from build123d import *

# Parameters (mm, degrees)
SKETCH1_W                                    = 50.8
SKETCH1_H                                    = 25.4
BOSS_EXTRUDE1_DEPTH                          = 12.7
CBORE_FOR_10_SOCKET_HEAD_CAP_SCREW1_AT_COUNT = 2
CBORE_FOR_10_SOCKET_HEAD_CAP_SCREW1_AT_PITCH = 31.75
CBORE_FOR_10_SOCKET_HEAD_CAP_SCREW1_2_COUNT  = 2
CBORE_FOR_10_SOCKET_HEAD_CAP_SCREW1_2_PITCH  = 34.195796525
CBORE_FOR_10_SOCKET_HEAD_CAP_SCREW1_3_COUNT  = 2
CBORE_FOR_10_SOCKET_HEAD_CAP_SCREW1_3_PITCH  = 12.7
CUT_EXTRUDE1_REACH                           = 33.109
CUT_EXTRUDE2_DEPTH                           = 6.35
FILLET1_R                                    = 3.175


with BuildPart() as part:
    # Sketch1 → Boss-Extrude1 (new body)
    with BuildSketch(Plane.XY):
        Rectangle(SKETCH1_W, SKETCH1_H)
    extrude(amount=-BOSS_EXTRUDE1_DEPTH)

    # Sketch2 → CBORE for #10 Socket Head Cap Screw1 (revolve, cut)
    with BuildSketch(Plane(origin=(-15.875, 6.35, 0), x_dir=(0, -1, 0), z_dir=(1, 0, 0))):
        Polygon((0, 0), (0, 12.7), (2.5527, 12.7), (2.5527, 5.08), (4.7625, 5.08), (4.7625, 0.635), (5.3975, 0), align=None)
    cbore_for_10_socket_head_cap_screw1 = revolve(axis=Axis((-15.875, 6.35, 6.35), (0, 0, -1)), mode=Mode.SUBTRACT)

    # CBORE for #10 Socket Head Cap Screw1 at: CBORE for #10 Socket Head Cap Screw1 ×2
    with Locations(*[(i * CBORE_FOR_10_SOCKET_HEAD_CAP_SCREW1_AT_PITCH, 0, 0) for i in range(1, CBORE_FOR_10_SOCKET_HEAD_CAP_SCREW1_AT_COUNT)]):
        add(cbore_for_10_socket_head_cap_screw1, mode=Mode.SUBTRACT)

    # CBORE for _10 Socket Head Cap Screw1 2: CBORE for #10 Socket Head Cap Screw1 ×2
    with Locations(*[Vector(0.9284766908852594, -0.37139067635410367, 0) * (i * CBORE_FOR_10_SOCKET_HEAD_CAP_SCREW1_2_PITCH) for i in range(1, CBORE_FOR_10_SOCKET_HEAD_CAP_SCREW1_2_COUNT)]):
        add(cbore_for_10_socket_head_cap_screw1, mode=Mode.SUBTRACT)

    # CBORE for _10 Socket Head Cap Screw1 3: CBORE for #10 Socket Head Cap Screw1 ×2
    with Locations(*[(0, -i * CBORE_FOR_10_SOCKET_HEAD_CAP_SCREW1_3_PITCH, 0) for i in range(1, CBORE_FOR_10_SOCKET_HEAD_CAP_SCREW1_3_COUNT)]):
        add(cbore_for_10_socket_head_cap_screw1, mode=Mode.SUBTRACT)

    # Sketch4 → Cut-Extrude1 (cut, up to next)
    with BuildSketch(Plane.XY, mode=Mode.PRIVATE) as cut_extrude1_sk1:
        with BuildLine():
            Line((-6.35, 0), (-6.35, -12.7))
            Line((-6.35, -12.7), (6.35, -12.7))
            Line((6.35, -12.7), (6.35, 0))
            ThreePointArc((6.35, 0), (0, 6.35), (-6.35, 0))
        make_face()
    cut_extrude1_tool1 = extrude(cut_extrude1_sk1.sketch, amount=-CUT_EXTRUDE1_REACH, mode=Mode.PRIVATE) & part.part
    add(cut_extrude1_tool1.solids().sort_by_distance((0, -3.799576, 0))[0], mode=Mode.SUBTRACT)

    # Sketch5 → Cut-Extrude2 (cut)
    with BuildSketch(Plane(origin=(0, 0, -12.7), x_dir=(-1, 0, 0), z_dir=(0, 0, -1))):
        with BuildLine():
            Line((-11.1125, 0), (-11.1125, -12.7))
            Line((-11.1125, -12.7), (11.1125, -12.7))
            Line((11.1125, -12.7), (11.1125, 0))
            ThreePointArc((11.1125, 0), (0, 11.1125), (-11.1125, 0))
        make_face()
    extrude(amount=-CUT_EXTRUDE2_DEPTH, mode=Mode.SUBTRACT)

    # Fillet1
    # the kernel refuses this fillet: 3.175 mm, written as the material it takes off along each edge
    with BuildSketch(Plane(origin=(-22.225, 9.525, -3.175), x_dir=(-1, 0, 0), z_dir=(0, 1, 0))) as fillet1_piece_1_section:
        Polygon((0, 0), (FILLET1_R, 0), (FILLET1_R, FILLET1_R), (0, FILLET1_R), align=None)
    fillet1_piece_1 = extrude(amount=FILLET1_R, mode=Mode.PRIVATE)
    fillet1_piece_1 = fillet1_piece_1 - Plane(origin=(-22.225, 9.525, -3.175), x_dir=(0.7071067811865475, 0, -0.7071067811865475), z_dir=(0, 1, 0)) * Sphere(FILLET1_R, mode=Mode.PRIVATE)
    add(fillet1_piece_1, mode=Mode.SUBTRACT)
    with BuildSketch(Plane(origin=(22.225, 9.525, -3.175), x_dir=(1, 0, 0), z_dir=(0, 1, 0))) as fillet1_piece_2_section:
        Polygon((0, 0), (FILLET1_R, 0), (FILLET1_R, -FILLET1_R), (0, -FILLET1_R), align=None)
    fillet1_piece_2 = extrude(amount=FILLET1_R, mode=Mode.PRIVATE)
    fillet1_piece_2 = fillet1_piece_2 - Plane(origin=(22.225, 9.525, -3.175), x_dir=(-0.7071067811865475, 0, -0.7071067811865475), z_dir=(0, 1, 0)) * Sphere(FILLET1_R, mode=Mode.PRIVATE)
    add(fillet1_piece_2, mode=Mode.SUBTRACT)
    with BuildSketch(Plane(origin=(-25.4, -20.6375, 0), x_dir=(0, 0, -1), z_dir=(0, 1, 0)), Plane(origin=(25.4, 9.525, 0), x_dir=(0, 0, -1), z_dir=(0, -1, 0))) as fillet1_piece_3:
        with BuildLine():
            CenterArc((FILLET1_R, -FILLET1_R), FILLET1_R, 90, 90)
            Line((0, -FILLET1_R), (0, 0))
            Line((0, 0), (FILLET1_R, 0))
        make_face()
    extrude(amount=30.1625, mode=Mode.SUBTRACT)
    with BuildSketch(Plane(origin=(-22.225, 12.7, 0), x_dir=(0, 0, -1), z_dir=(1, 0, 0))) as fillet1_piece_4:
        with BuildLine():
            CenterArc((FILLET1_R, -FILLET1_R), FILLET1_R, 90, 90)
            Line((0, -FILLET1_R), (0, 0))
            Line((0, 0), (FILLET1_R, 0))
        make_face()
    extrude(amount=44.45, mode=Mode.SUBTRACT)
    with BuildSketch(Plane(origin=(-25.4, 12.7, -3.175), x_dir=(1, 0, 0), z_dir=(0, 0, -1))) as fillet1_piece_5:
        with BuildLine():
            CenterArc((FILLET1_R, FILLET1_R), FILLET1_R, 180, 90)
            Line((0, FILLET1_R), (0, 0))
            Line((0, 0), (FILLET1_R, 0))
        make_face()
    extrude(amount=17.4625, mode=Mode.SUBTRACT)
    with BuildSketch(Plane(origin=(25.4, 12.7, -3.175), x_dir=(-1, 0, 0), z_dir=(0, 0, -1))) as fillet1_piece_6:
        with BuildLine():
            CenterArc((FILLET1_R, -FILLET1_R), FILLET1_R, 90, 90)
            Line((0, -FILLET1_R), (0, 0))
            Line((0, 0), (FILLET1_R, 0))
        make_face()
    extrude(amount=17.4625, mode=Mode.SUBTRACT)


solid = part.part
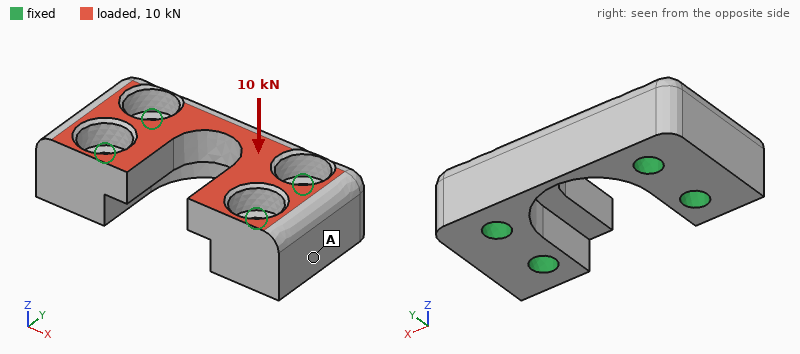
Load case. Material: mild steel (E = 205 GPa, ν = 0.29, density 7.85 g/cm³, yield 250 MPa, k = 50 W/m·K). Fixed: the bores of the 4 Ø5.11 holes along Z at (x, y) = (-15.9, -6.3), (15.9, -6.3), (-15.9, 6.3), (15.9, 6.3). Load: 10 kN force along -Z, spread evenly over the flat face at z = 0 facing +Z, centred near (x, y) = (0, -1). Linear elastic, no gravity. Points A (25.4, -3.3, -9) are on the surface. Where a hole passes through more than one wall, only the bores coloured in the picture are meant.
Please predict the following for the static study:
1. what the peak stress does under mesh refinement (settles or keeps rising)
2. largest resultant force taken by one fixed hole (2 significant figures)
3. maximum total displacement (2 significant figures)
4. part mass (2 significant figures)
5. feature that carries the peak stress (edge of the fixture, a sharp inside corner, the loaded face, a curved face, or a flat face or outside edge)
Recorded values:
keeps rising
2.8 kN
9.6 µm
75 g
edge of the fixture
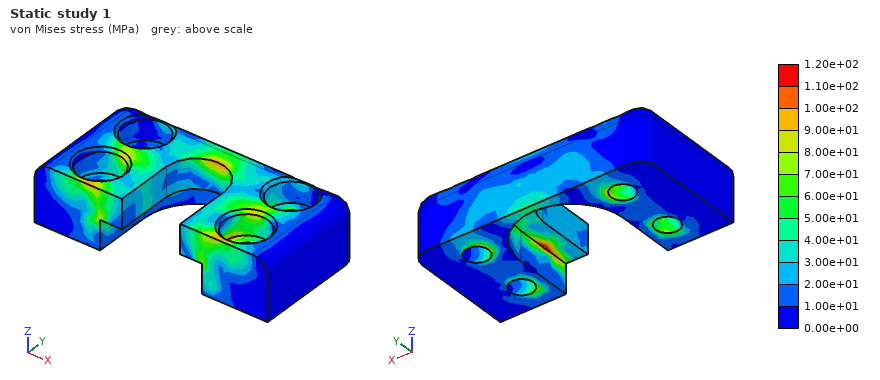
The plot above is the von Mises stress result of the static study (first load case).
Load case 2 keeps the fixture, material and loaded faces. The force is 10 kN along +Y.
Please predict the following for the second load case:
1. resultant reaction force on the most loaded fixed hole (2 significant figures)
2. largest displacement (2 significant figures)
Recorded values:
3.5 kN
9.7 µm
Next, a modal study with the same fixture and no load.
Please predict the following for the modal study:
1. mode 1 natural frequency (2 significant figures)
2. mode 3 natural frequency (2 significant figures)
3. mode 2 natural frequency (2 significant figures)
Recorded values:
35 kHz
41 kHz
38 kHz
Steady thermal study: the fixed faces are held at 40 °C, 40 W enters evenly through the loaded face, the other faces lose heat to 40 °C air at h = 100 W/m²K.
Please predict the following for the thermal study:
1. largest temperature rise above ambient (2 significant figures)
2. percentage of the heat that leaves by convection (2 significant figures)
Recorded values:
22 K
7.3 %
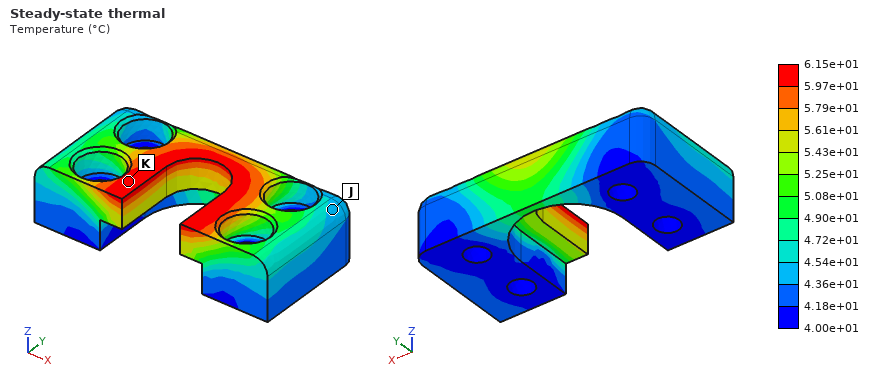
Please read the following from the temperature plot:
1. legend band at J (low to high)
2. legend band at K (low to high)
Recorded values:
4.36e+01 to 4.54e+01 °C
5.97e+01 to 6.15e+01 °C
